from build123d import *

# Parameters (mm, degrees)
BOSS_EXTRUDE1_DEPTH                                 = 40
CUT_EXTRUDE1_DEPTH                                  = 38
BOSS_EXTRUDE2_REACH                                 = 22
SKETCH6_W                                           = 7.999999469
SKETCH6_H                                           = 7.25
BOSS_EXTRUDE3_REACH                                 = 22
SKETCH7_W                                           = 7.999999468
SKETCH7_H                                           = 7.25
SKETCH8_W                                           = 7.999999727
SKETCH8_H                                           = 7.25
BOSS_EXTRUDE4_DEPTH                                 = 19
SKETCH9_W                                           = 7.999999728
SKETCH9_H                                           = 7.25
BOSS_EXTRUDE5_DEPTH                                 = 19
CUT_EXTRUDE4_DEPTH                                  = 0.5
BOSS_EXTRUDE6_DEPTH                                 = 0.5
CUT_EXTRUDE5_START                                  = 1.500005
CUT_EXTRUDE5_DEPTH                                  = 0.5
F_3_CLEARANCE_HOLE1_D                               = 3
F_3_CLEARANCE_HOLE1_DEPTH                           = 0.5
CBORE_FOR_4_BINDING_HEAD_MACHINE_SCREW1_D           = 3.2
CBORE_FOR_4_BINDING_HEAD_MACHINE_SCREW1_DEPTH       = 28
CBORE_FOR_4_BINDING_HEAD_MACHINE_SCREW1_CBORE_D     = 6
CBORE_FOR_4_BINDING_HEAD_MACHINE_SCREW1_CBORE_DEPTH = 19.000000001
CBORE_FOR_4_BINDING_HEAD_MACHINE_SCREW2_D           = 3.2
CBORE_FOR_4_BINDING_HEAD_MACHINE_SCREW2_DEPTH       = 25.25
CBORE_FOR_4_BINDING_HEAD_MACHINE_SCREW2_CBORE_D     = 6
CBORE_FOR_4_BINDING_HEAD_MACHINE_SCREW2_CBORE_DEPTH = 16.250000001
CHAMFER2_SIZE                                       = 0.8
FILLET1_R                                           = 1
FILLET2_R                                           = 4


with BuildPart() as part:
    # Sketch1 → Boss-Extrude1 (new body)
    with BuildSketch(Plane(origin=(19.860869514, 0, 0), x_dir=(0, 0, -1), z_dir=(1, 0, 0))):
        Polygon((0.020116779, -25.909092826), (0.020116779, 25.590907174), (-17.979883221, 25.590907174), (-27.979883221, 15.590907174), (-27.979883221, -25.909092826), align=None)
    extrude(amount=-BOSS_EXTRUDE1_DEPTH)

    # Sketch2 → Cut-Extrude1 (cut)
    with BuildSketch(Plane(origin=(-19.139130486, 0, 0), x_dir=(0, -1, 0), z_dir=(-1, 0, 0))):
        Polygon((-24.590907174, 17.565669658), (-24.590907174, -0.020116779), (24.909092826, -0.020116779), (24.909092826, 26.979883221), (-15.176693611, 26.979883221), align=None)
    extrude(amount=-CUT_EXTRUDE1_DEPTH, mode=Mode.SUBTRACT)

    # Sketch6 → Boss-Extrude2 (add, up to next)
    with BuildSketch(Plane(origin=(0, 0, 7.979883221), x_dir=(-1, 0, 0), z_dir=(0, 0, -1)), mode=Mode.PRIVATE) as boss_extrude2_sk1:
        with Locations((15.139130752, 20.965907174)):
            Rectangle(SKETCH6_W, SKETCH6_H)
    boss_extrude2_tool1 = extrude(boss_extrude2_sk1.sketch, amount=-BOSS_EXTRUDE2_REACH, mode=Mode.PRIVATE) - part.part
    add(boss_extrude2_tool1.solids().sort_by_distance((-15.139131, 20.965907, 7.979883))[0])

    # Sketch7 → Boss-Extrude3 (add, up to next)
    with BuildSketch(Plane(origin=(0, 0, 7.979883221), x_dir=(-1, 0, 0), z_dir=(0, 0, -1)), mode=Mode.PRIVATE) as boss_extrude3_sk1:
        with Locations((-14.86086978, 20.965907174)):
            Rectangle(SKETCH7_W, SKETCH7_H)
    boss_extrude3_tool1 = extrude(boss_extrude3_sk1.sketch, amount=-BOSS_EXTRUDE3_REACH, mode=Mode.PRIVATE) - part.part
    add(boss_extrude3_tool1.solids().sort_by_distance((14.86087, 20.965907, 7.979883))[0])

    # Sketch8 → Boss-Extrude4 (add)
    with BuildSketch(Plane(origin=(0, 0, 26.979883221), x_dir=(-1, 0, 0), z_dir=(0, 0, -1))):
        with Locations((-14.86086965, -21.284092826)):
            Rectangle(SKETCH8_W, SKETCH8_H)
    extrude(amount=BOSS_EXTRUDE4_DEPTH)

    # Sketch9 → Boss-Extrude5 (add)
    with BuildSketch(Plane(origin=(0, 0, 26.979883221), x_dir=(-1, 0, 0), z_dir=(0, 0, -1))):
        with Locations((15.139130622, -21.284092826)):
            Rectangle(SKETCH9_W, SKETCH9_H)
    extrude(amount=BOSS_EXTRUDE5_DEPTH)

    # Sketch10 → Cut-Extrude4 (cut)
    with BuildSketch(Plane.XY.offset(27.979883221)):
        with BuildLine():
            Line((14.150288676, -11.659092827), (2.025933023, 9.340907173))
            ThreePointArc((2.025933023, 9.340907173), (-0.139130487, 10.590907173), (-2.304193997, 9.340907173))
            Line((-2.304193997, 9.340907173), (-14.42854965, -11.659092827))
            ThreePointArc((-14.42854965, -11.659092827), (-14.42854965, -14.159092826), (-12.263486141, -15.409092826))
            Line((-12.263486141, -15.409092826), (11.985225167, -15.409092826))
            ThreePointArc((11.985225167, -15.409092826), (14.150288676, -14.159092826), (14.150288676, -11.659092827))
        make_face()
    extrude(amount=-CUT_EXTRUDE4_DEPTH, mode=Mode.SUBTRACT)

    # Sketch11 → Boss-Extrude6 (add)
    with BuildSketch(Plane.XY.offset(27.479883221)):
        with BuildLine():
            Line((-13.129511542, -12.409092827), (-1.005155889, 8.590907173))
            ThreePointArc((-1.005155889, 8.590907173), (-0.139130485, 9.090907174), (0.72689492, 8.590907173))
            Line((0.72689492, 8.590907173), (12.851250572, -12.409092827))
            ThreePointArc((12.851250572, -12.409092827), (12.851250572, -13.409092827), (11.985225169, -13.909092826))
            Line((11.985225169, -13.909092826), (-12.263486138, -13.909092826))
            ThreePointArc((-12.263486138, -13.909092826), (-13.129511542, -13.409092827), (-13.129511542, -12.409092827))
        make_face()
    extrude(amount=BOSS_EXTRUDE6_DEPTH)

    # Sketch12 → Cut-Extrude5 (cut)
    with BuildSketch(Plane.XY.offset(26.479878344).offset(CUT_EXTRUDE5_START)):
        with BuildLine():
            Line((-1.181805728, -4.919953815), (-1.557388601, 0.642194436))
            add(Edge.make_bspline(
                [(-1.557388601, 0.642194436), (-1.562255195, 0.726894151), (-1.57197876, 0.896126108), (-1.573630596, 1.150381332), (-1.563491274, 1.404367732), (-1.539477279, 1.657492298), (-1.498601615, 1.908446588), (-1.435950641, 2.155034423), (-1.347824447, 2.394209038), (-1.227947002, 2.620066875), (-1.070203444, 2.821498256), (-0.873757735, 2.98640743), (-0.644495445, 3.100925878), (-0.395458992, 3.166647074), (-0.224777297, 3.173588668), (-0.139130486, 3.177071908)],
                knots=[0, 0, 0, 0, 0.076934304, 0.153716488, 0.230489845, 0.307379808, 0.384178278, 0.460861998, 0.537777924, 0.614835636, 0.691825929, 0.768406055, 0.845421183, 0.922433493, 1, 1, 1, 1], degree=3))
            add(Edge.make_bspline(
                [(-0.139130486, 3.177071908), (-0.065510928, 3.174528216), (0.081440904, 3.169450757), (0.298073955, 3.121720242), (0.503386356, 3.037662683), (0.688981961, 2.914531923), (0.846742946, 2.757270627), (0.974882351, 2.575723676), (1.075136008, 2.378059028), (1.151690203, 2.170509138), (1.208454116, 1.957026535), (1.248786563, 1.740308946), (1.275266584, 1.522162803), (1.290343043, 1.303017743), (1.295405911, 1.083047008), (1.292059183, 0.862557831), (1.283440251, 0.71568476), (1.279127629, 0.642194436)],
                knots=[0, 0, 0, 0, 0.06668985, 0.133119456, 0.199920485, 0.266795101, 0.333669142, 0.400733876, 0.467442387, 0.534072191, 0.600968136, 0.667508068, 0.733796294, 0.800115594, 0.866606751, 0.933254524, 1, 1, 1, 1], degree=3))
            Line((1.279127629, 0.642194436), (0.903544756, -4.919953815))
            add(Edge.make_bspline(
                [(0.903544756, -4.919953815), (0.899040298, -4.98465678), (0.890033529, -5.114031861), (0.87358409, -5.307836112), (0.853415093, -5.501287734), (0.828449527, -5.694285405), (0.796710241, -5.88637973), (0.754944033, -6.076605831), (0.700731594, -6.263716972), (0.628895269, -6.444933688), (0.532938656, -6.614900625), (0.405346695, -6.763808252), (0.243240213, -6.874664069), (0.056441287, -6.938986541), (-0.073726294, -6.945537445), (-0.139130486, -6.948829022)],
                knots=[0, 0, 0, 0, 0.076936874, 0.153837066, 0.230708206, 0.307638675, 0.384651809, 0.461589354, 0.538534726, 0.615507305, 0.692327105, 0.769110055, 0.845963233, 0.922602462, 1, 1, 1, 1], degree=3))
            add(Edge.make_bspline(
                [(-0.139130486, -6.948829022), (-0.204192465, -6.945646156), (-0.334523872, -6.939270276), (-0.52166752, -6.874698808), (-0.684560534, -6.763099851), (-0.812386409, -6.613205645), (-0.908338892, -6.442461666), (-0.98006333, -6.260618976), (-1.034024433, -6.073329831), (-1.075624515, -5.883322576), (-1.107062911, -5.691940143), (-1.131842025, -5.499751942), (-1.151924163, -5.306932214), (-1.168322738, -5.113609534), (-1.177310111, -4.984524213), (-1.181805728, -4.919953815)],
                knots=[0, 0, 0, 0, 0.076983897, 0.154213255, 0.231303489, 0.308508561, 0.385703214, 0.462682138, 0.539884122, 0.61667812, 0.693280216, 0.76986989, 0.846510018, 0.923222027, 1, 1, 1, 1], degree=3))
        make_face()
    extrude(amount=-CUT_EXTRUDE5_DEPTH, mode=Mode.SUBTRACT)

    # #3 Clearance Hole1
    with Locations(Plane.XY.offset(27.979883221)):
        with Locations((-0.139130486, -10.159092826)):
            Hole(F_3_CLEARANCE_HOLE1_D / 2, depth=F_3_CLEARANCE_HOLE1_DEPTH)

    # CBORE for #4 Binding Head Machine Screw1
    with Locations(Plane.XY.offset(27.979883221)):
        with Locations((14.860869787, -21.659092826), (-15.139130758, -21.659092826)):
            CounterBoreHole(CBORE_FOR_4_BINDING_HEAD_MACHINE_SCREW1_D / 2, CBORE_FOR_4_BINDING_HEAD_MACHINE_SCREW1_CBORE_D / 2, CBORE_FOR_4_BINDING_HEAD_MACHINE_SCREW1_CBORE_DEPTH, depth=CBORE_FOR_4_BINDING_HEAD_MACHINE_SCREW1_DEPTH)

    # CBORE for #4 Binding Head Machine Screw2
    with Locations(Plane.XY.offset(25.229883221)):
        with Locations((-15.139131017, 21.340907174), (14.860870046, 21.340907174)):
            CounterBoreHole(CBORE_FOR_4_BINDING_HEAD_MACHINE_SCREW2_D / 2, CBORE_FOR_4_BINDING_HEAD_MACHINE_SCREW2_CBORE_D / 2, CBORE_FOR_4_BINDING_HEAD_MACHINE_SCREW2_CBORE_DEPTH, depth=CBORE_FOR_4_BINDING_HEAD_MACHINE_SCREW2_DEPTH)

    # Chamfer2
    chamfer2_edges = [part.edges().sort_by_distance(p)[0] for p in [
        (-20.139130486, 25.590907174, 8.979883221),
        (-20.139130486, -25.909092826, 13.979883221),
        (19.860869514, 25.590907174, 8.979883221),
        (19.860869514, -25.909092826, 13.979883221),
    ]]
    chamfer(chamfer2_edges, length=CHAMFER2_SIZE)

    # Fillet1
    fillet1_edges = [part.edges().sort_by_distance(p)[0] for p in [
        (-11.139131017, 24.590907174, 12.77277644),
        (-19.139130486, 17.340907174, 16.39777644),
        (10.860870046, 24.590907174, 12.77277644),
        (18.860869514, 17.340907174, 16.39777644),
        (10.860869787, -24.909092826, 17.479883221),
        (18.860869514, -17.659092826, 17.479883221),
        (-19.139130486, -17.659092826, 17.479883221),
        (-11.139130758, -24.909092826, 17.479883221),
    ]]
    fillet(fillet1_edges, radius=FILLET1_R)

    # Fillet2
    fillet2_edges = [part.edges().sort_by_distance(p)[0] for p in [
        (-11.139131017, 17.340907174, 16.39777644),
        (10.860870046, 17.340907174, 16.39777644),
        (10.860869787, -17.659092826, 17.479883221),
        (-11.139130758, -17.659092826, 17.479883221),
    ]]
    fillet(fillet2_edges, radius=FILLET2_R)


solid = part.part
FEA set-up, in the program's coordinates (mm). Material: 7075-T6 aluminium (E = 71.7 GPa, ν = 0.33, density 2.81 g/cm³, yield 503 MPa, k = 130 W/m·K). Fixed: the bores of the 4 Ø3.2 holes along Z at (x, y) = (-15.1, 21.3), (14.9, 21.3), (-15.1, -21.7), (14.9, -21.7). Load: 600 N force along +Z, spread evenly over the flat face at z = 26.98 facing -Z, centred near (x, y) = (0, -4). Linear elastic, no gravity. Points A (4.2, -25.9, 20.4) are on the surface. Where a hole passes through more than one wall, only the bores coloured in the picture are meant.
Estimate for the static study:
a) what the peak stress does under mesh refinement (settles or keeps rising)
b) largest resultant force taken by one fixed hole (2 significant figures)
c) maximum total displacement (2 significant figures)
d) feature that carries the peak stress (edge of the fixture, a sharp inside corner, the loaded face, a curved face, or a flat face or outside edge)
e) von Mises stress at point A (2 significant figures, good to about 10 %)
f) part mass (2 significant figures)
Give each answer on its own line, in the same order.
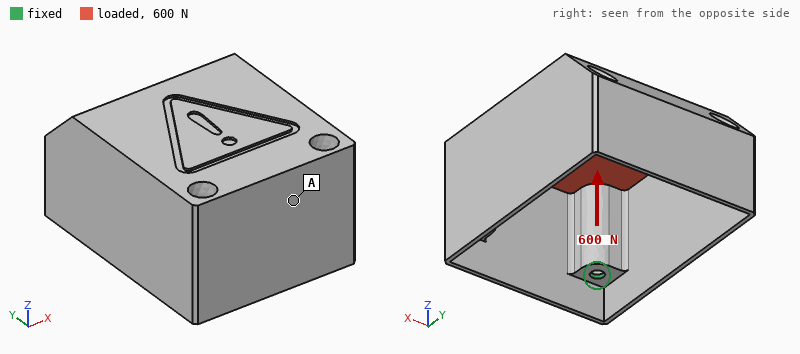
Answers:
keeps rising
180 N
0.32 mm
a sharp inside corner
14 MPa
23 g
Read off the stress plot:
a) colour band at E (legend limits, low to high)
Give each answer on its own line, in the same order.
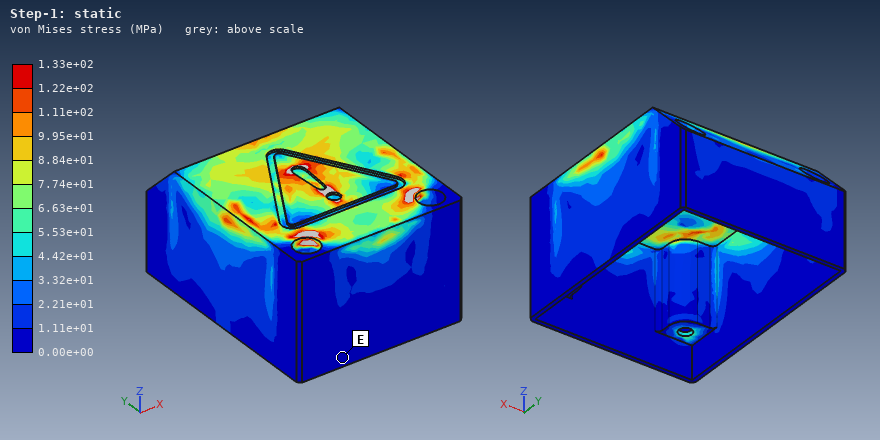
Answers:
0.00e+00 to 1.11e+01 MPa
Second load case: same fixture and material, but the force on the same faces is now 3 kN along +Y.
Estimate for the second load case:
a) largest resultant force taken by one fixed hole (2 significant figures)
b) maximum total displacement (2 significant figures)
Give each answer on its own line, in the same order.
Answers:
980 N
80 µm
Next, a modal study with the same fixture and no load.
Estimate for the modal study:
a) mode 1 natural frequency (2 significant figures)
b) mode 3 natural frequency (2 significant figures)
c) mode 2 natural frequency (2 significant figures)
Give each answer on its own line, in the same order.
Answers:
4000 Hz
4700 Hz
4000 Hz
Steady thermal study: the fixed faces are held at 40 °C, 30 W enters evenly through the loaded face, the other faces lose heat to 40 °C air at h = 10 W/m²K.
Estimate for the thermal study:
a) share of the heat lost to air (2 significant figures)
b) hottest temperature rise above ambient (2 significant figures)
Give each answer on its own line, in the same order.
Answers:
8.2 %
50 K
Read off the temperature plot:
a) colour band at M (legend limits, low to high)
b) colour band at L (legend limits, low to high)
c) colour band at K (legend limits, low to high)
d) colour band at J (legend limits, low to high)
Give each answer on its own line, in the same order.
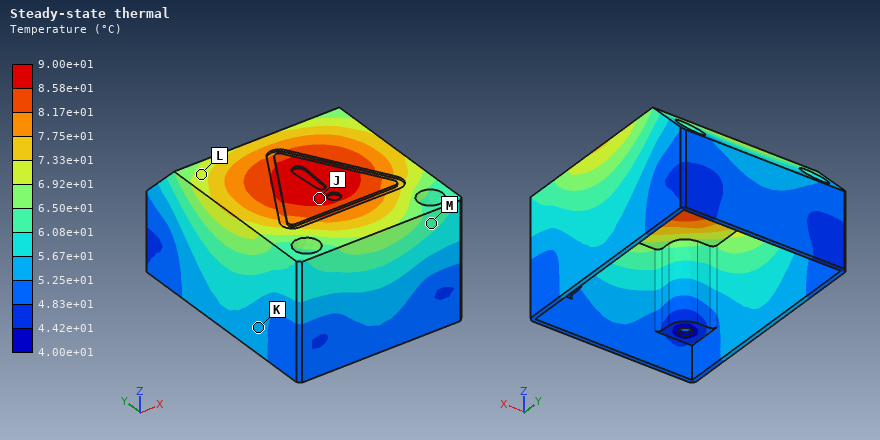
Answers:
6.08e+01 to 6.50e+01 °C
6.92e+01 to 7.33e+01 °C
5.25e+01 to 5.67e+01 °C
8.58e+01 to 9.00e+01 °C
